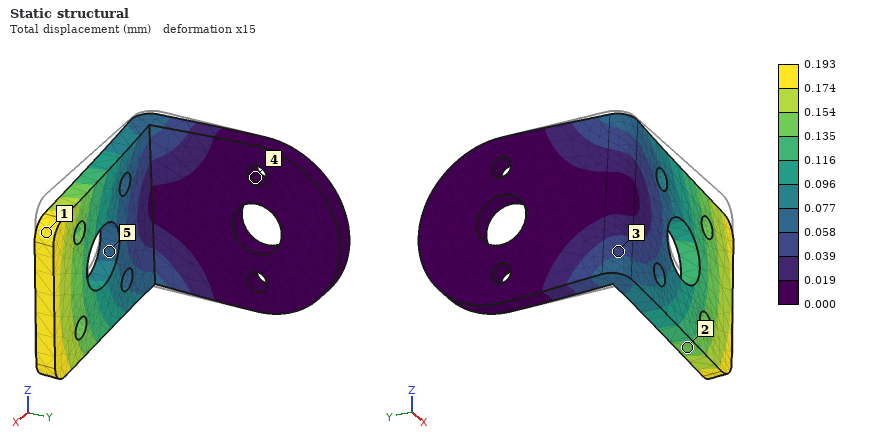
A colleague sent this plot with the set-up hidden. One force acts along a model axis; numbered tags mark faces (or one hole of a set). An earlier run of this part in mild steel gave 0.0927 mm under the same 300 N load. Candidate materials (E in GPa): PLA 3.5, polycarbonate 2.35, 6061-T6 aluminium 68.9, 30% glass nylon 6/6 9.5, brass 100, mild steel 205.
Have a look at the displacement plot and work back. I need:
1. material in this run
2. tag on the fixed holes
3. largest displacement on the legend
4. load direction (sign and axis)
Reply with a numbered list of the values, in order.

1. brass
2. 4
3. 0.193 mm
4. -Z
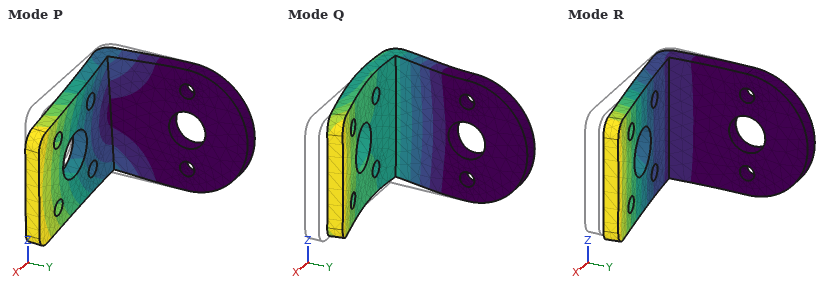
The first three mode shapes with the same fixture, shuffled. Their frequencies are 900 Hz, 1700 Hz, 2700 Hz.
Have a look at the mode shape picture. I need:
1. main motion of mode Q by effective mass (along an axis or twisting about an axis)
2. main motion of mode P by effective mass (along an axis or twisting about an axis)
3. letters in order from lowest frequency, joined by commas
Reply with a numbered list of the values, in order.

1. along X
2. along Z
3. R, P, Q
